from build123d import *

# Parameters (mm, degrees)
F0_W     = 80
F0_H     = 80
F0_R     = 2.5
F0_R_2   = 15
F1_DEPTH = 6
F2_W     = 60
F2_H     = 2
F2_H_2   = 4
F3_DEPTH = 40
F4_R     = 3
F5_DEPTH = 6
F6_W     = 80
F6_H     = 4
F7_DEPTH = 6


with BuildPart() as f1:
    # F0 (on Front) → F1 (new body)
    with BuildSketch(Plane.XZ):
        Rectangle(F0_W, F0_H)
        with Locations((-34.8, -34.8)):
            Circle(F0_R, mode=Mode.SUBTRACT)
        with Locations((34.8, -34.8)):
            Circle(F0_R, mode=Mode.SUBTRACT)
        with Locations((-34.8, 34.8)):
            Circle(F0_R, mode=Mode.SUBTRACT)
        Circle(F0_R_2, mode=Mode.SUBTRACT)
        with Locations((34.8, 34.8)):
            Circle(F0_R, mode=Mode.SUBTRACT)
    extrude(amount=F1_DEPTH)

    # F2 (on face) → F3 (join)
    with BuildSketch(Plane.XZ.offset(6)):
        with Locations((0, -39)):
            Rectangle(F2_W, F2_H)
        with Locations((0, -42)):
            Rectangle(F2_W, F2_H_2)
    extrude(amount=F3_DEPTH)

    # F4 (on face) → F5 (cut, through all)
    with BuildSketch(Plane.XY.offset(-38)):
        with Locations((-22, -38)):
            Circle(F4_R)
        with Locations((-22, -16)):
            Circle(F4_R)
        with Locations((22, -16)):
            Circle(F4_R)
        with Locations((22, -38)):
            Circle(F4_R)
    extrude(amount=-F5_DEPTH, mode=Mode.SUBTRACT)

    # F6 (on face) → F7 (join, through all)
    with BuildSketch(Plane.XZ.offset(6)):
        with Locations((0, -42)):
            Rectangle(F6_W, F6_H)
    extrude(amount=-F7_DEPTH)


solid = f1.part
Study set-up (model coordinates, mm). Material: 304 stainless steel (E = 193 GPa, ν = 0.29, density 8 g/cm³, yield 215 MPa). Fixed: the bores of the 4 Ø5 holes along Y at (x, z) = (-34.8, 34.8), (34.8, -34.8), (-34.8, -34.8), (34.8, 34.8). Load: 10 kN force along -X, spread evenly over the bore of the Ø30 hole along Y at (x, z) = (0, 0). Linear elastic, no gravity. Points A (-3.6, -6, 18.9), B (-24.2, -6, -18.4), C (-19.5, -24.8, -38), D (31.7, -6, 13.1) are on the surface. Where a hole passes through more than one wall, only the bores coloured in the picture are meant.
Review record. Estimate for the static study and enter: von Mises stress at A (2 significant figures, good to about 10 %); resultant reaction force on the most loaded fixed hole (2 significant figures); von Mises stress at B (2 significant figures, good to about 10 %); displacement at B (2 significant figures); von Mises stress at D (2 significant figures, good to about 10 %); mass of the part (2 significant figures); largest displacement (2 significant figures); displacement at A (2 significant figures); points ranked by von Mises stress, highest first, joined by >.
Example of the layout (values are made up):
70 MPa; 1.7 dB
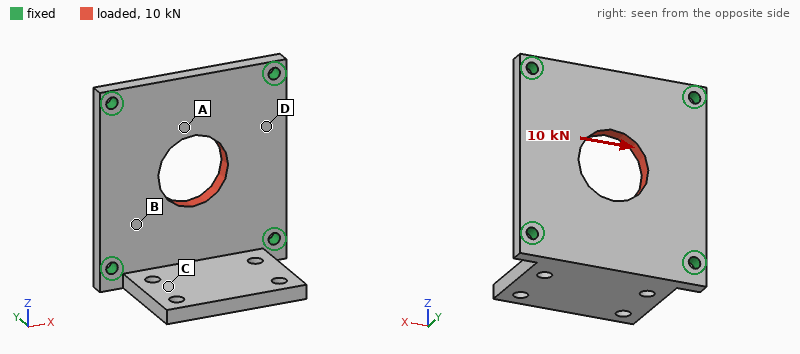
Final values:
28 MPa; 2.8 kN; 21 MPa; 3.7 µm; 11 MPa; 390 g; 6.6 µm; 4.3 µm; A > B > D > C
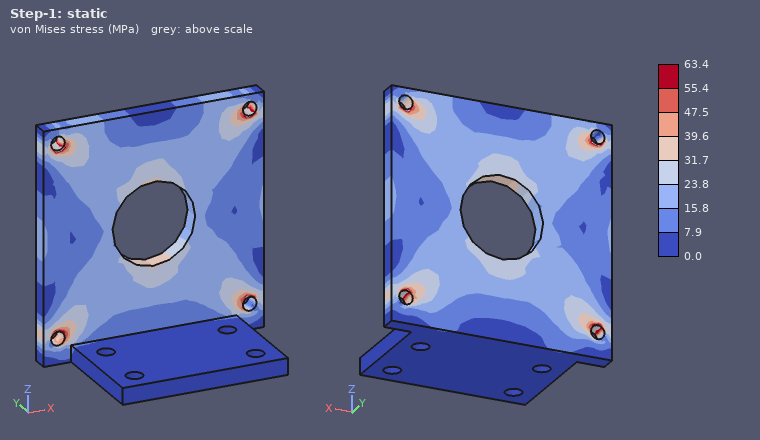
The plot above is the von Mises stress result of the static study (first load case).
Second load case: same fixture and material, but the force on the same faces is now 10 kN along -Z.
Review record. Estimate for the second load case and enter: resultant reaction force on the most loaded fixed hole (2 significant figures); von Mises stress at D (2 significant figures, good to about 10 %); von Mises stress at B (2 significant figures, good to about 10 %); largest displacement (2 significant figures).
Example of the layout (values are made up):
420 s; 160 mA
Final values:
2.7 kN; 14 MPa; 20 MPa; 6.7 µm
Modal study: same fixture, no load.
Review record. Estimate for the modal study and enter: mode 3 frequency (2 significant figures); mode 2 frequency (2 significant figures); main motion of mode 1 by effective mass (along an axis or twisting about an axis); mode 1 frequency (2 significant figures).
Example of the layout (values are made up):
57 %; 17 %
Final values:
4600 Hz; 4500 Hz; along Z; 1900 Hz
